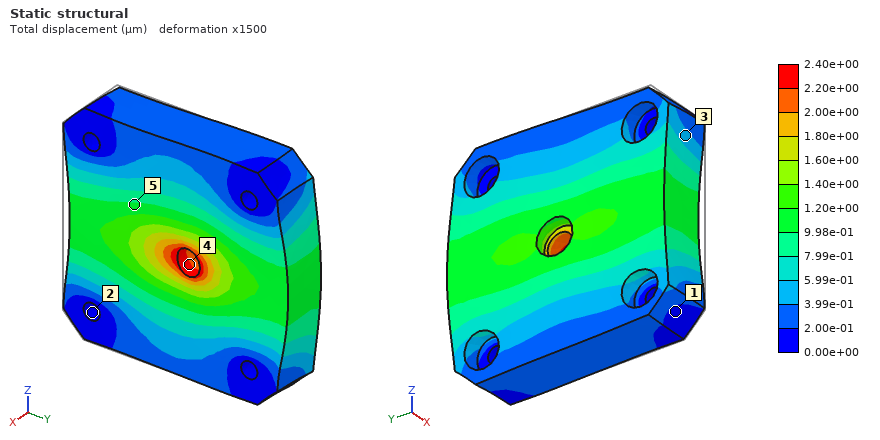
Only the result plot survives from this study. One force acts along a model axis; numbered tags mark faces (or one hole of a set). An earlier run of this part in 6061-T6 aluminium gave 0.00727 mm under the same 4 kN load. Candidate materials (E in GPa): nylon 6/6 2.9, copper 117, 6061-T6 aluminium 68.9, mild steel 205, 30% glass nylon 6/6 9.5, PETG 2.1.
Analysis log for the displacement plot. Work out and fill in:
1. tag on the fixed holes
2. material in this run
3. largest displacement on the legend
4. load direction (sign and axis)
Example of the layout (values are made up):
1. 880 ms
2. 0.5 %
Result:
1. 2
2. mild steel
3. 2.40e+00 µm
4. +Y
